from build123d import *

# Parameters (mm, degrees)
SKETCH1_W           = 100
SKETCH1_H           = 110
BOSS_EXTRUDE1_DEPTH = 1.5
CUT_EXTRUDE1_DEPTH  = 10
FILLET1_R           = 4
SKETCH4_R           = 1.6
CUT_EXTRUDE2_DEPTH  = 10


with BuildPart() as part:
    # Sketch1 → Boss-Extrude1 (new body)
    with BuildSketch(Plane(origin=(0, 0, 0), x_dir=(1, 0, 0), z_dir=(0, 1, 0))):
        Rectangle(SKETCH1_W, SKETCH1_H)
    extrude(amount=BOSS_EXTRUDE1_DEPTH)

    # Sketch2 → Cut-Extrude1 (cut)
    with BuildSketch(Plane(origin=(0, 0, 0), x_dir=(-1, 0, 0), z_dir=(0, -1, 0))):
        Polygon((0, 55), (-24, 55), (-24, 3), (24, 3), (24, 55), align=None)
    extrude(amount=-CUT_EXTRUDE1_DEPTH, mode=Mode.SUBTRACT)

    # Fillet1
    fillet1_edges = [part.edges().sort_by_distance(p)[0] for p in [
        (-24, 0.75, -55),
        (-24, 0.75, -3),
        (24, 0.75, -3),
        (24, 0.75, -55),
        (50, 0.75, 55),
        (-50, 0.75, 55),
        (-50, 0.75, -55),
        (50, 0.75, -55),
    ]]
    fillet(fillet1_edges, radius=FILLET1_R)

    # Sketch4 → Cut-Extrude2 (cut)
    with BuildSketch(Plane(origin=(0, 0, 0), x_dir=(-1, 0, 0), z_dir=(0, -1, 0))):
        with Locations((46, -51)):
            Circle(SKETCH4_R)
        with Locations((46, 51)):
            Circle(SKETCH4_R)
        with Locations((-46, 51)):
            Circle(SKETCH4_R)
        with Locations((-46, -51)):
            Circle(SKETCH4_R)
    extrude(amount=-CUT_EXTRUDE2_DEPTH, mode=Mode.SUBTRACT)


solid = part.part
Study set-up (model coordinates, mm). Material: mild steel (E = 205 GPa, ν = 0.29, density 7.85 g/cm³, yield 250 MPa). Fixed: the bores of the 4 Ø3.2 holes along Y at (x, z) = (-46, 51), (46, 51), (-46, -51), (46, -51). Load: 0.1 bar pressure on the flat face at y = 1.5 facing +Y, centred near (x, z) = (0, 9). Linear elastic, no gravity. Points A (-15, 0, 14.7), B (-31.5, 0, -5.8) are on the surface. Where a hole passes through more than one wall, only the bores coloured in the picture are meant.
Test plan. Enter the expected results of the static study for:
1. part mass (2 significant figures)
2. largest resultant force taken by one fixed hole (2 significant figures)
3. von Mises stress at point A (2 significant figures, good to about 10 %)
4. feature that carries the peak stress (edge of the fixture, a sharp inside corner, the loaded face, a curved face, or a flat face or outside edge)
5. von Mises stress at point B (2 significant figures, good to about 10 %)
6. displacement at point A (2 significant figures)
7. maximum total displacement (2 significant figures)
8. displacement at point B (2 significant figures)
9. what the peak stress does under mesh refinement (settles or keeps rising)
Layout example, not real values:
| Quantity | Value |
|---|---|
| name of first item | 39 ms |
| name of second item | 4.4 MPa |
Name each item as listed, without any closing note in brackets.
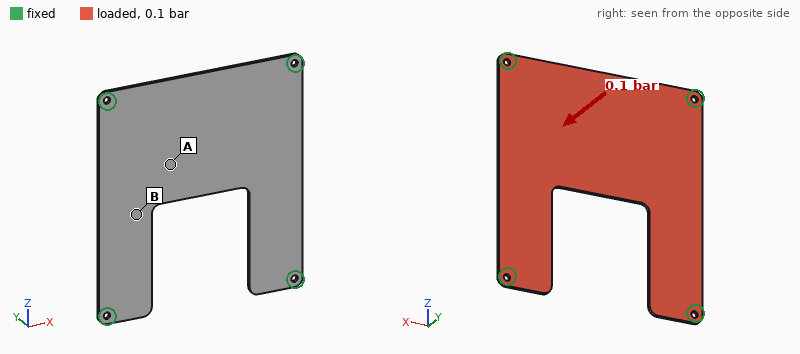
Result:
| Quantity | Value |
|---|---|
| part mass | 100 g |
| largest resultant force taken by one fixed hole | 25 N |
| von Mises stress at point A | 10 MPa |
| feature that carries the peak stress | edge of the fixture |
| von Mises stress at point B | 20 MPa |
| displacement at point A | 0.11 mm |
| maximum total displacement | 0.14 mm |
| displacement at point B | 0.10 mm |
| what the peak stress does under mesh refinement | keeps rising |
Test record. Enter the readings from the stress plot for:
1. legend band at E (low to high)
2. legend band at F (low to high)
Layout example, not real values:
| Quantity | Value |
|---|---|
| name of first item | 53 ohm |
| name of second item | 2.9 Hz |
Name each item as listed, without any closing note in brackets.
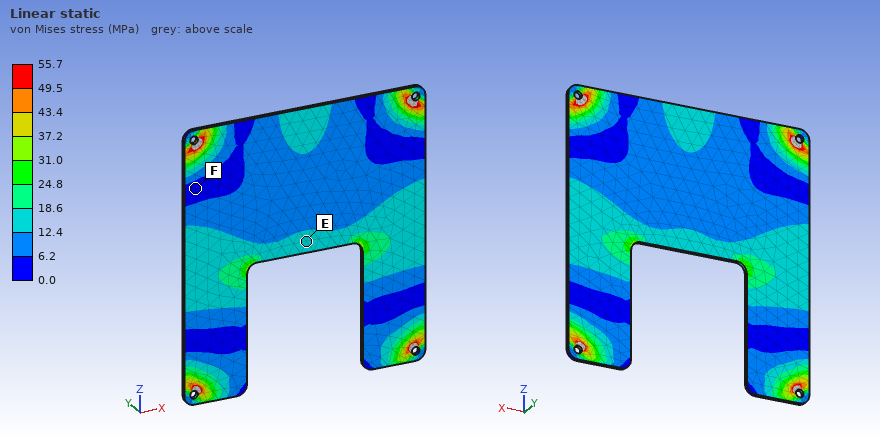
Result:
| Quantity | Value |
|---|---|
| legend band at E | 12.4 to 18.6 MPa |
| legend band at F | 0.0 to 6.2 MPa |
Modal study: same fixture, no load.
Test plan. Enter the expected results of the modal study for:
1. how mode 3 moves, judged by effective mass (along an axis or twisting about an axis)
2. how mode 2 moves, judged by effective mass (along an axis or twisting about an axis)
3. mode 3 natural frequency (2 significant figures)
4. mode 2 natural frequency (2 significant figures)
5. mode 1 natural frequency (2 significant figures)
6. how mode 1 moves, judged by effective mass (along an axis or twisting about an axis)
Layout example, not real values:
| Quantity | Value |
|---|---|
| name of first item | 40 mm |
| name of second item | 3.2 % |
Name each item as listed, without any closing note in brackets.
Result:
| Quantity | Value |
|---|---|
| how mode 3 moves, judged by effective mass | twisting about X |
| how mode 2 moves, judged by effective mass | twisting about Z |
| mode 3 natural frequency | 980 Hz |
| mode 2 natural frequency | 810 Hz |
| mode 1 natural frequency | 500 Hz |
| how mode 1 moves, judged by effective mass | along Y |
